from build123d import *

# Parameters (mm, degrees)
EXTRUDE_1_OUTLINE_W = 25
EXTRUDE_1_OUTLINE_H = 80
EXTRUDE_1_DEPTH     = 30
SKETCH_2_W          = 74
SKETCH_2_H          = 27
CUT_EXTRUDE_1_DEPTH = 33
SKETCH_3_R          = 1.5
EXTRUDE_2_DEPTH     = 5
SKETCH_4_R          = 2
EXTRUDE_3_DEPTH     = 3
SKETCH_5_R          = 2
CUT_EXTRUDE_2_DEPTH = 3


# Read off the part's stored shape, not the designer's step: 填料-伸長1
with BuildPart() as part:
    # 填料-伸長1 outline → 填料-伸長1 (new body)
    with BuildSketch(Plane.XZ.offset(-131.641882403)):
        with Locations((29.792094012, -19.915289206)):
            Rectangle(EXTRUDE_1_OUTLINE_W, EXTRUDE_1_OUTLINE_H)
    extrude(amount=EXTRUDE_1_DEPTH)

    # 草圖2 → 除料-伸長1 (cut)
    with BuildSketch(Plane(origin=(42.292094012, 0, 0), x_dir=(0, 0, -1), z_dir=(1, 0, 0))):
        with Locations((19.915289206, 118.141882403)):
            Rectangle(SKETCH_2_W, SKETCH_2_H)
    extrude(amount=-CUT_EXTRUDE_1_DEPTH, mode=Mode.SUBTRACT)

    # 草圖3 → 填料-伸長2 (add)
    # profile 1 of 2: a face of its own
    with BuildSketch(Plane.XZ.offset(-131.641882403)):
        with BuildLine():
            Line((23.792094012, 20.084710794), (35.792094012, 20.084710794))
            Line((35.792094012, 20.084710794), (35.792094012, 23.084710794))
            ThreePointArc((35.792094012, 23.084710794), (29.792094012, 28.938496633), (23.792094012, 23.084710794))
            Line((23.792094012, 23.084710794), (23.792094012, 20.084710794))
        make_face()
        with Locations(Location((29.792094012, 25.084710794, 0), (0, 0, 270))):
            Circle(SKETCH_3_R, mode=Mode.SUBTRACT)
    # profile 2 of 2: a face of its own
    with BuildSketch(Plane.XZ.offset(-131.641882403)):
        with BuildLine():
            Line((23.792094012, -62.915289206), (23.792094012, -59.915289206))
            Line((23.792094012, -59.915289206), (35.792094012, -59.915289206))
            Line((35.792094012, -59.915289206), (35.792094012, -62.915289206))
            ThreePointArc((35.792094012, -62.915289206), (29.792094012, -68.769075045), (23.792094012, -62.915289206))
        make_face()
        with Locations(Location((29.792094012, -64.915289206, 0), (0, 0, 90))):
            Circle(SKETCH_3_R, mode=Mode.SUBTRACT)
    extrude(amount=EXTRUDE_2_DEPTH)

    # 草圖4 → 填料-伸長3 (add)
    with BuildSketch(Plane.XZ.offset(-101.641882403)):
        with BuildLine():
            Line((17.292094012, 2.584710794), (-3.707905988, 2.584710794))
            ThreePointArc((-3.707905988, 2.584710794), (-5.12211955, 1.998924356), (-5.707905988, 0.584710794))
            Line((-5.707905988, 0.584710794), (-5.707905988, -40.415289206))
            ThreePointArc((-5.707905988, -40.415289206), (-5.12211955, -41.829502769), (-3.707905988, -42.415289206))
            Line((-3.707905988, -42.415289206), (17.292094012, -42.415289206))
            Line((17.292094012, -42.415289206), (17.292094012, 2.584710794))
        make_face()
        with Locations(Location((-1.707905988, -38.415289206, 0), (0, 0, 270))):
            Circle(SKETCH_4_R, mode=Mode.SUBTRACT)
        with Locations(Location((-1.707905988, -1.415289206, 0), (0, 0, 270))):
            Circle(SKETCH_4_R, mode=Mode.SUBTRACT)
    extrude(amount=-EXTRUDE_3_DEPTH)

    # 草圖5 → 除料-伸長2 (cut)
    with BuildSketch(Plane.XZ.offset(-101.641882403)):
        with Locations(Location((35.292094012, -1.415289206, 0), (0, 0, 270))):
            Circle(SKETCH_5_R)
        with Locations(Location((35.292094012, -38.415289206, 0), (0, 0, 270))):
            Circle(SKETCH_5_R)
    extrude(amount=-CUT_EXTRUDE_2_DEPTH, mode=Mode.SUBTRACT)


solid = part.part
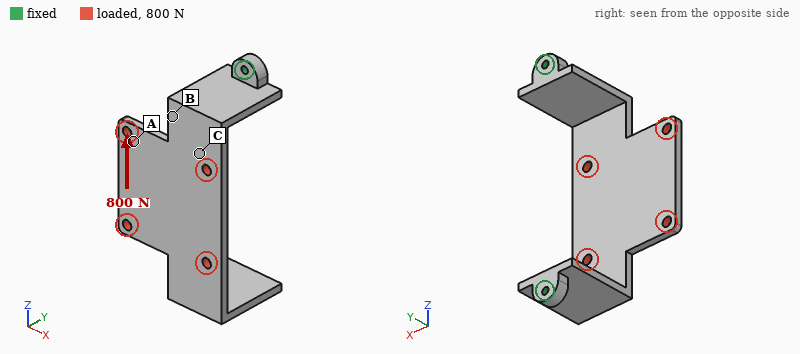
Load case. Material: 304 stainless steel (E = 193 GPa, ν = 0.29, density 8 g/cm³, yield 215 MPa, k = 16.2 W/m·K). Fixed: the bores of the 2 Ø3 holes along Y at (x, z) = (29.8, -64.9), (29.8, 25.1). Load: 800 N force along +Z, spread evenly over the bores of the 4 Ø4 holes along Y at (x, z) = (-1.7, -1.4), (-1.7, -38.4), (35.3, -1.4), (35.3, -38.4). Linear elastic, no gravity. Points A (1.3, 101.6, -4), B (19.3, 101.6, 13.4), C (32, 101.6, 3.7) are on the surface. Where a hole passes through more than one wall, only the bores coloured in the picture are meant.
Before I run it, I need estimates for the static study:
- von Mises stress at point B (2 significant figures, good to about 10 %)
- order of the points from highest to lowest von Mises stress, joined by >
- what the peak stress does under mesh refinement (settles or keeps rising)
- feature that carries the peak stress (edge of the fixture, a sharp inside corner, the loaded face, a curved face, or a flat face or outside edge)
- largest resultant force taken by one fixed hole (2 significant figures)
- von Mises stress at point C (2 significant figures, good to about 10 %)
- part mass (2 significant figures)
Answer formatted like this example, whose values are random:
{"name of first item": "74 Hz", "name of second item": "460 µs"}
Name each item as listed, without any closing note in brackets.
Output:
{"von Mises stress at point B": "93 MPa", "order of the points from highest to lowest von Mises stress, joined by >": "B > C > A", "what the peak stress does under mesh refinement": "keeps rising", "feature that carries the peak stress": "edge of the fixture", "largest resultant force taken by one fixed hole": "430 N", "von Mises stress at point C": "57 MPa", "part mass": "110 g"}
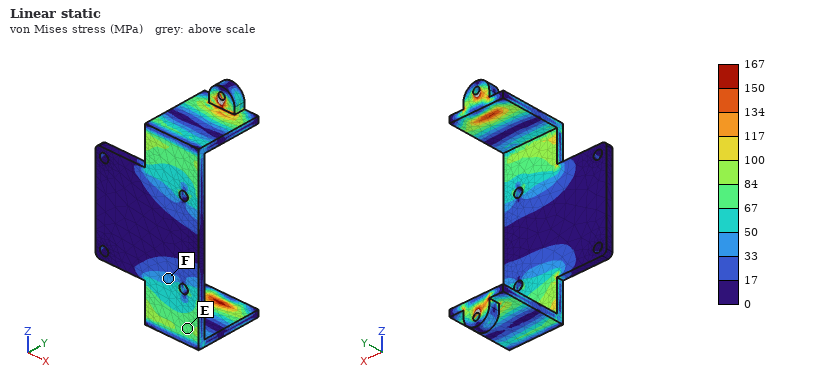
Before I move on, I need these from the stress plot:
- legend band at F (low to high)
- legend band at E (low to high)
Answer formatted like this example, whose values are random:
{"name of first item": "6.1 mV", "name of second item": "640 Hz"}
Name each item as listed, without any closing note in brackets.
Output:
{"legend band at F": "33 to 50 MPa", "legend band at E": "67 to 84 MPa"}
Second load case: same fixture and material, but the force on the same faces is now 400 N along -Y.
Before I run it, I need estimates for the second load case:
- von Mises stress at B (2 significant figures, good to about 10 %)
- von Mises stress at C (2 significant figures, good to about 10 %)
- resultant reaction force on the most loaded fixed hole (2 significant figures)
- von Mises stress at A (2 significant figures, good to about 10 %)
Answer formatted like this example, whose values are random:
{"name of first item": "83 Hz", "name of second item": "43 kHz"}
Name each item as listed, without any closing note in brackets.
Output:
{"von Mises stress at B": "79 MPa", "von Mises stress at C": "38 MPa", "resultant reaction force on the most loaded fixed hole": "240 N", "von Mises stress at A": "36 MPa"}
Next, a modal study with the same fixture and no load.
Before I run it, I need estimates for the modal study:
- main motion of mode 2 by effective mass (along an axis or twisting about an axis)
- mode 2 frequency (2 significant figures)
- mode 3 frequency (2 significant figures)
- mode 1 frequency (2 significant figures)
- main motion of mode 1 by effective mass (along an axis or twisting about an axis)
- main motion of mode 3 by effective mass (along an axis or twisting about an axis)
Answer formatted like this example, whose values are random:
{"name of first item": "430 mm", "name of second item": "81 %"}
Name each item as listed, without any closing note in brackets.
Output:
{"main motion of mode 2 by effective mass": "along Z", "mode 2 frequency": "1400 Hz", "mode 3 frequency": "2000 Hz", "mode 1 frequency": "1200 Hz", "main motion of mode 1 by effective mass": "along Y", "main motion of mode 3 by effective mass": "along X"}
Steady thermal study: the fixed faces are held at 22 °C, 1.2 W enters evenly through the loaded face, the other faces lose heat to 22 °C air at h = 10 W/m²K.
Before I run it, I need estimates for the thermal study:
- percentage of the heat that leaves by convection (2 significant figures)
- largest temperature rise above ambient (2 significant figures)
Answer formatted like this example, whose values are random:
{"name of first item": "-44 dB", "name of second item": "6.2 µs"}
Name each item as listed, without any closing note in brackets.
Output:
{"percentage of the heat that leaves by convection": "66 %", "largest temperature rise above ambient": "18 K"}
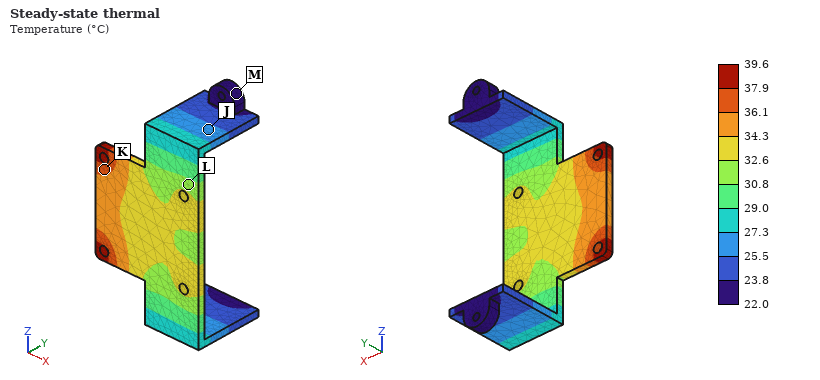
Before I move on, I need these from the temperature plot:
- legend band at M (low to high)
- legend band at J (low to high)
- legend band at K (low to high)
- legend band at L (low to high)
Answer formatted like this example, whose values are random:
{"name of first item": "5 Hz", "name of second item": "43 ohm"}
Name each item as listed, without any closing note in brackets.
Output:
{"legend band at M": "22.0 to 23.8 °C", "legend band at J": "25.5 to 27.3 °C", "legend band at K": "36.1 to 37.9 °C", "legend band at L": "30.8 to 32.6 °C"}
